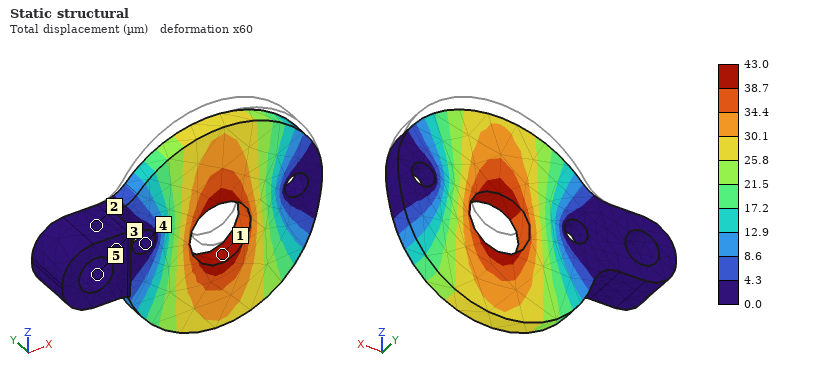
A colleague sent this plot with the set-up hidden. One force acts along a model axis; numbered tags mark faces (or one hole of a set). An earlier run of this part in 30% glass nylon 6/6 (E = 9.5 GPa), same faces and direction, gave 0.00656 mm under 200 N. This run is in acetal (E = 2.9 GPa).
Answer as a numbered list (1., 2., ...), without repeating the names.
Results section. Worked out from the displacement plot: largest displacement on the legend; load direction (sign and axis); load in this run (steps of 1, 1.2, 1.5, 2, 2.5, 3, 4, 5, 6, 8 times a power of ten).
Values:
1. 43.0 µm
2. -Z
3. 400 N
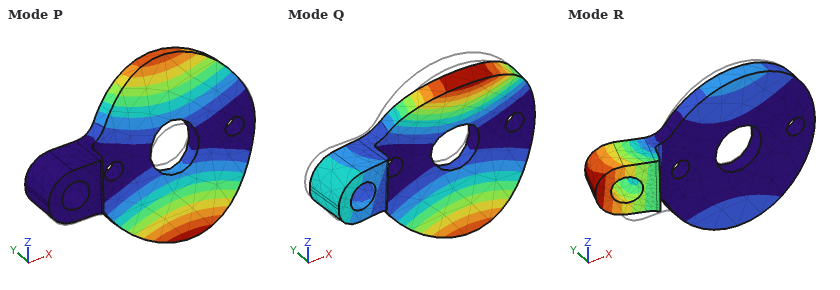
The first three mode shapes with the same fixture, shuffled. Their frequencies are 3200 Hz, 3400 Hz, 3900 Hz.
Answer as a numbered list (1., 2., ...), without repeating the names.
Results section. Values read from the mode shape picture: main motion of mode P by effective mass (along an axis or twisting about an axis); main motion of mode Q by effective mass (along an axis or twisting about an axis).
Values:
1. twisting about X
2. along Y
